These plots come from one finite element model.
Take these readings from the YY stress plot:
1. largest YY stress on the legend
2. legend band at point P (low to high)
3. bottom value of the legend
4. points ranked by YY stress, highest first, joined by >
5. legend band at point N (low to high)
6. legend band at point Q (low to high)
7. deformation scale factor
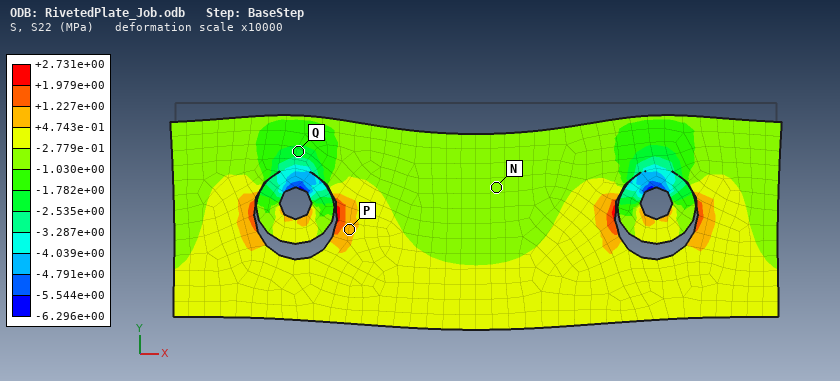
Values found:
+2.731e+00 MPa
+4.743e-01 to +1.227e+00 MPa
-6.296e+00 MPa
P > N > Q
-1.030e+00 to -2.779e-01 MPa
-2.535e+00 to -1.782e+00 MPa
10000
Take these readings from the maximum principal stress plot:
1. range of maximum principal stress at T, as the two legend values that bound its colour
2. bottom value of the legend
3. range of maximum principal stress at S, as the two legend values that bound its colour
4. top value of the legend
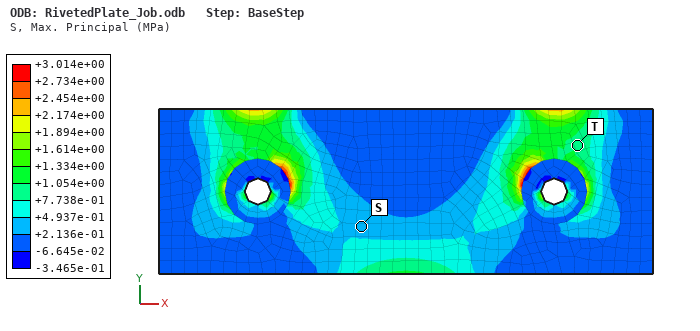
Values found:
+7.738e-01 to +1.054e+00 MPa
-3.465e-01 MPa
+2.136e-01 to +4.937e-01 MPa
+3.014e+00 MPa
